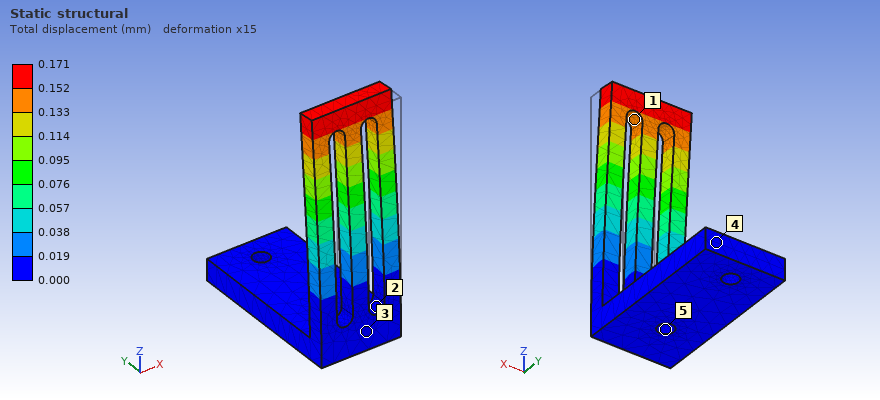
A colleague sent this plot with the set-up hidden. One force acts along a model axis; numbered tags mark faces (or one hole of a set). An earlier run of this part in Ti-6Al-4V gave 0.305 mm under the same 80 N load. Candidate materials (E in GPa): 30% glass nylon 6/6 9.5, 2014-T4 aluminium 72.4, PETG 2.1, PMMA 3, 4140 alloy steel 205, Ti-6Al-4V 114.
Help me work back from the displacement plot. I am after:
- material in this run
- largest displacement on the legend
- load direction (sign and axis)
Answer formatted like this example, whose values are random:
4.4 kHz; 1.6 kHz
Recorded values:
4140 alloy steel; 0.171 mm; +Y
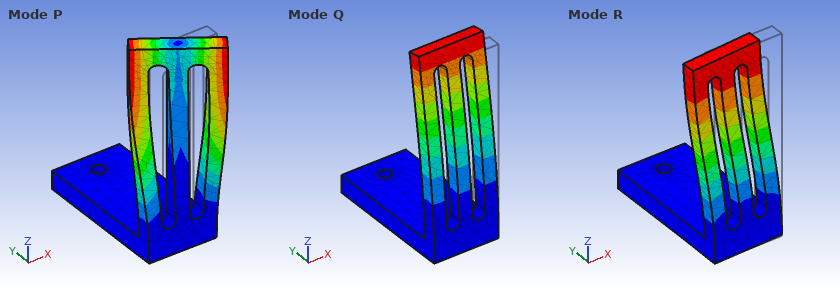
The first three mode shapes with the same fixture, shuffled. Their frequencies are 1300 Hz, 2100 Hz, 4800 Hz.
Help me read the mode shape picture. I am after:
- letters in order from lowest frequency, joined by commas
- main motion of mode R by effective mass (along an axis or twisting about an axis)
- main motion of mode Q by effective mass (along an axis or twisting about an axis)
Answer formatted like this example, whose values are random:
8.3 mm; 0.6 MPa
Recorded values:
Q, R, P; along X; along Y
